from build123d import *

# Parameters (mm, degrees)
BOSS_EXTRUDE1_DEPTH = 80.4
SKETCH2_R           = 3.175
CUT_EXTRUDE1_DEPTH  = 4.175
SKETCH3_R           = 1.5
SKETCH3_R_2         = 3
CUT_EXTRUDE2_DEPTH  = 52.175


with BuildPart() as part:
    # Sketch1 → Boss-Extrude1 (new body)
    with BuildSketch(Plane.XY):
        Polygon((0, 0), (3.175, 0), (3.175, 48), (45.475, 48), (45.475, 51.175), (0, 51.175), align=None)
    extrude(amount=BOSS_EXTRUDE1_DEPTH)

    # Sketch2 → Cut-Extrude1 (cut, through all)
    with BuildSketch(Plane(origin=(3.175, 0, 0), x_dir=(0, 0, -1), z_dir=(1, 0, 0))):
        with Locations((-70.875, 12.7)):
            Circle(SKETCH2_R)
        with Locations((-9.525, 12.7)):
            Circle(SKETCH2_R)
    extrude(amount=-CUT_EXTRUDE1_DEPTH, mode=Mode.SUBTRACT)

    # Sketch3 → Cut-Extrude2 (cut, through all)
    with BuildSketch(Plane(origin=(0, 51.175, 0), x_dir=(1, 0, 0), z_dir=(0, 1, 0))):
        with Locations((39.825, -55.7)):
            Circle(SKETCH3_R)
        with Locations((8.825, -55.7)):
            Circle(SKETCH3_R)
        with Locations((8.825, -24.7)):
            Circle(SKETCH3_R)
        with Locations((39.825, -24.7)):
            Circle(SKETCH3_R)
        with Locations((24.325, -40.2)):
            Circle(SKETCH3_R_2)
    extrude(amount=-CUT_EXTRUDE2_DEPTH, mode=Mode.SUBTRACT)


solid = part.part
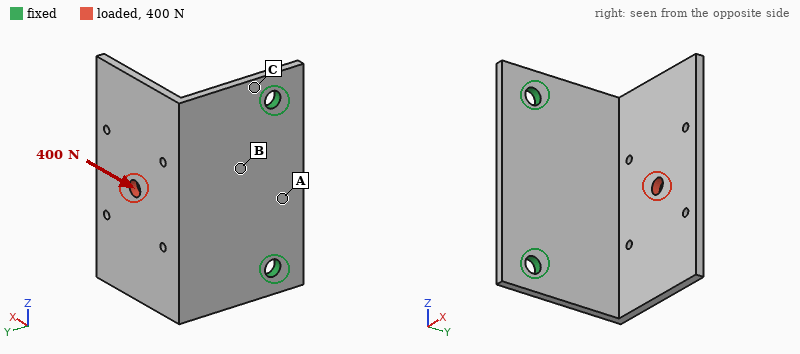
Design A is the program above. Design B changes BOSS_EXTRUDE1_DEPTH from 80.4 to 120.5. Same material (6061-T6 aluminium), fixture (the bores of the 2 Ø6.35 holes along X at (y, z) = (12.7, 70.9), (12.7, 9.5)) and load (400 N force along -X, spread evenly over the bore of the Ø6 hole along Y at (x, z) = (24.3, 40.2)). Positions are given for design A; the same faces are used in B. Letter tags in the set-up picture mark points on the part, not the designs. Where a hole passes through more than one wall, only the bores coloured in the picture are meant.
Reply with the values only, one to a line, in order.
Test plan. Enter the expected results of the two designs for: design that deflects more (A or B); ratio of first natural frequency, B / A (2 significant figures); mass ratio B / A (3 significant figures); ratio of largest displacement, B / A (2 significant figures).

A
0.91
1.51
0.86
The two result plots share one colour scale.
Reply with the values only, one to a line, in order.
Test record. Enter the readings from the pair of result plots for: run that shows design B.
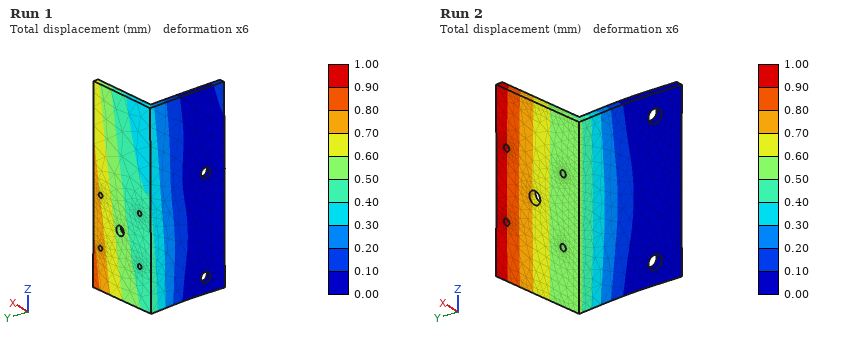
Run 1
